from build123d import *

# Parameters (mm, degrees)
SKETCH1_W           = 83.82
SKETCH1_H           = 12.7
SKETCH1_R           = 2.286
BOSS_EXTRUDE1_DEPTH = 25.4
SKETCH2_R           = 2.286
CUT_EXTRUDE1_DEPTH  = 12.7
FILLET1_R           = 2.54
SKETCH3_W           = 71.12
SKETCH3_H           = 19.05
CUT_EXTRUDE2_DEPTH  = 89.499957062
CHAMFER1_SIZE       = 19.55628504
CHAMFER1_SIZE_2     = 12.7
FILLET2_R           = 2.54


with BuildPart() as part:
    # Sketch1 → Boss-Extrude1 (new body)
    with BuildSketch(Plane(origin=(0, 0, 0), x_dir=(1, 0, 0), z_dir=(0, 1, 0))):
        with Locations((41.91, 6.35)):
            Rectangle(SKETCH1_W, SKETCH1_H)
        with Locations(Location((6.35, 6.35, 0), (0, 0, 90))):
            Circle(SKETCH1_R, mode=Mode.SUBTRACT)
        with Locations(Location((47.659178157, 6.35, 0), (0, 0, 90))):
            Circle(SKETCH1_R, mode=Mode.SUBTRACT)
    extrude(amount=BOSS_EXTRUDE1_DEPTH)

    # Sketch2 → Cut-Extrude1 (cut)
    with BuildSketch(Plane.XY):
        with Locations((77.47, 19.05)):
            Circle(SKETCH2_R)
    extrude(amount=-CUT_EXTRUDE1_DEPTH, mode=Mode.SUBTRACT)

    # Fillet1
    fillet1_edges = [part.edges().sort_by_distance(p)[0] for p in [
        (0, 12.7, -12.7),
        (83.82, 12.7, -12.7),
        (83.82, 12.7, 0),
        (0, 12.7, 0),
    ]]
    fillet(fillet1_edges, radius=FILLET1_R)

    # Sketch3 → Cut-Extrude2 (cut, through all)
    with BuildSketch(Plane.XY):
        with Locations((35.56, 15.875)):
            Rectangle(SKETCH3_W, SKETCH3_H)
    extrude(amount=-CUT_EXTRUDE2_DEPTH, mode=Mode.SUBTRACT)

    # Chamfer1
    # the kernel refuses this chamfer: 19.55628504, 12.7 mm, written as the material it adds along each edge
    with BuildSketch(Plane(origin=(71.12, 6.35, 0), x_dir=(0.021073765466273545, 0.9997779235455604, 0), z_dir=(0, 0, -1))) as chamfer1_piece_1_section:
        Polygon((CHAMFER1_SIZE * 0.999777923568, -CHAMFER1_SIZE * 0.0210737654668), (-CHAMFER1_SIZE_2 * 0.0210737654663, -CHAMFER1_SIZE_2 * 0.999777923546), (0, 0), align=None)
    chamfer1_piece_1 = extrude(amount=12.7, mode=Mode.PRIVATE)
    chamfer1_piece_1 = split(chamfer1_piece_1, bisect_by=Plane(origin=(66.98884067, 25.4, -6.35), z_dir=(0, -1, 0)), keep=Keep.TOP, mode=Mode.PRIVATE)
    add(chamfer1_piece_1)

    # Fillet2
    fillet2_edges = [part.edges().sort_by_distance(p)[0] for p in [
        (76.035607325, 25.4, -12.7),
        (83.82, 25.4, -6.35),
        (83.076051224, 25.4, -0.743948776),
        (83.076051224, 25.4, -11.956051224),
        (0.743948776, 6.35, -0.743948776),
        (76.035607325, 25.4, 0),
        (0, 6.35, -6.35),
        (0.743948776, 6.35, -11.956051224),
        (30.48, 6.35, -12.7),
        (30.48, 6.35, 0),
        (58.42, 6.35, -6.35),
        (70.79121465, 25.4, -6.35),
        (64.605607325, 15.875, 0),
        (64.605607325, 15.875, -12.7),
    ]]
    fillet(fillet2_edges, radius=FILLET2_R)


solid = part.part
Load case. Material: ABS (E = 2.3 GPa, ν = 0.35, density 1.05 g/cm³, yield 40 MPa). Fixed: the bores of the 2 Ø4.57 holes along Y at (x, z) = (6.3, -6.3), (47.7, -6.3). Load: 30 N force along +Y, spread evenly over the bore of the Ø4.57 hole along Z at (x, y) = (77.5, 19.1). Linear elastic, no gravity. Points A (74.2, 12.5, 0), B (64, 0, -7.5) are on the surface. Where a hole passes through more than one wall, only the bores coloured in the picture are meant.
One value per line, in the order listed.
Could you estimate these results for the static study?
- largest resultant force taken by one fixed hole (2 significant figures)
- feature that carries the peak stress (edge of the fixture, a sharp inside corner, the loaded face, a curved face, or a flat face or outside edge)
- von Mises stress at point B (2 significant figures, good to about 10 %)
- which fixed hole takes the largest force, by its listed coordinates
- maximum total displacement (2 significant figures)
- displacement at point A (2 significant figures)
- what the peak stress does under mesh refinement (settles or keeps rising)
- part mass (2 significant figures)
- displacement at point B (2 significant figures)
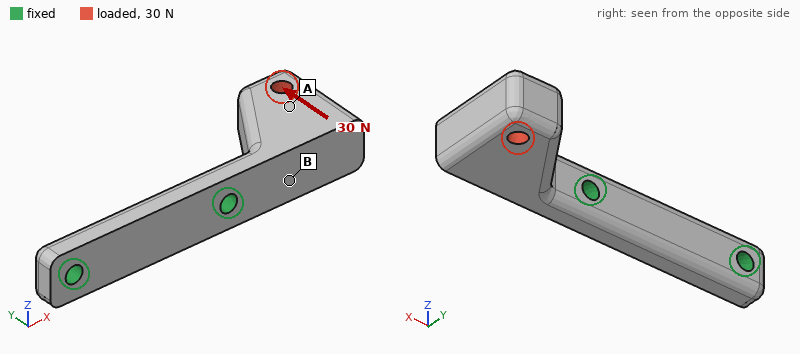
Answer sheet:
31 N
edge of the fixture
2.2 MPa
(47.7, -6.3)
0.54 mm
0.33 mm
keeps rising
11 g
0.15 mm
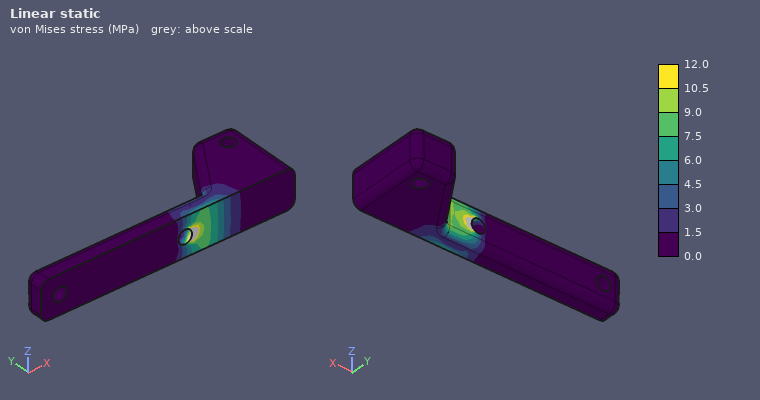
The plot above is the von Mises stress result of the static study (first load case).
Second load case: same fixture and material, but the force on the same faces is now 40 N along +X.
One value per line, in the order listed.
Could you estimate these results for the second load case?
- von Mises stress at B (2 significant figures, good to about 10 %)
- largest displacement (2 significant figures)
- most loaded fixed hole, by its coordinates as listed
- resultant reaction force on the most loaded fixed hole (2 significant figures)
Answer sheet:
2.5 MPa
0.50 mm
(47.7, -6.3)
40 N
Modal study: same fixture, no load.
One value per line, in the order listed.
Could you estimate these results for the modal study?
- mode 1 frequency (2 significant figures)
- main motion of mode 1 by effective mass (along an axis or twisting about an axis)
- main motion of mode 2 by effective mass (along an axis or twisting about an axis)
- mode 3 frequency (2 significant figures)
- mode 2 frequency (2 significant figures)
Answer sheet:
600 Hz
along Y
along Z
2000 Hz
870 Hz
